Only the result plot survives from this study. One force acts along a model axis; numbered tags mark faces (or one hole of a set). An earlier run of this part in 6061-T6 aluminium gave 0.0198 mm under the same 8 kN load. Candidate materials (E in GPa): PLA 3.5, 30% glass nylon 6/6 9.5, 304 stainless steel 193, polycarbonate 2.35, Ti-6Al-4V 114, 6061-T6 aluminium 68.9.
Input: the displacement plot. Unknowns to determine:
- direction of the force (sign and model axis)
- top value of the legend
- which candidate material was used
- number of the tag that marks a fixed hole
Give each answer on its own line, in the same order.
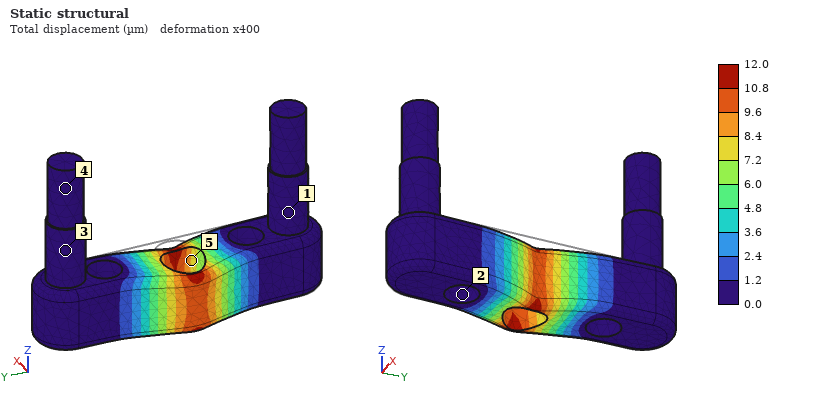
-X
12.0 µm
Ti-6Al-4V
2
